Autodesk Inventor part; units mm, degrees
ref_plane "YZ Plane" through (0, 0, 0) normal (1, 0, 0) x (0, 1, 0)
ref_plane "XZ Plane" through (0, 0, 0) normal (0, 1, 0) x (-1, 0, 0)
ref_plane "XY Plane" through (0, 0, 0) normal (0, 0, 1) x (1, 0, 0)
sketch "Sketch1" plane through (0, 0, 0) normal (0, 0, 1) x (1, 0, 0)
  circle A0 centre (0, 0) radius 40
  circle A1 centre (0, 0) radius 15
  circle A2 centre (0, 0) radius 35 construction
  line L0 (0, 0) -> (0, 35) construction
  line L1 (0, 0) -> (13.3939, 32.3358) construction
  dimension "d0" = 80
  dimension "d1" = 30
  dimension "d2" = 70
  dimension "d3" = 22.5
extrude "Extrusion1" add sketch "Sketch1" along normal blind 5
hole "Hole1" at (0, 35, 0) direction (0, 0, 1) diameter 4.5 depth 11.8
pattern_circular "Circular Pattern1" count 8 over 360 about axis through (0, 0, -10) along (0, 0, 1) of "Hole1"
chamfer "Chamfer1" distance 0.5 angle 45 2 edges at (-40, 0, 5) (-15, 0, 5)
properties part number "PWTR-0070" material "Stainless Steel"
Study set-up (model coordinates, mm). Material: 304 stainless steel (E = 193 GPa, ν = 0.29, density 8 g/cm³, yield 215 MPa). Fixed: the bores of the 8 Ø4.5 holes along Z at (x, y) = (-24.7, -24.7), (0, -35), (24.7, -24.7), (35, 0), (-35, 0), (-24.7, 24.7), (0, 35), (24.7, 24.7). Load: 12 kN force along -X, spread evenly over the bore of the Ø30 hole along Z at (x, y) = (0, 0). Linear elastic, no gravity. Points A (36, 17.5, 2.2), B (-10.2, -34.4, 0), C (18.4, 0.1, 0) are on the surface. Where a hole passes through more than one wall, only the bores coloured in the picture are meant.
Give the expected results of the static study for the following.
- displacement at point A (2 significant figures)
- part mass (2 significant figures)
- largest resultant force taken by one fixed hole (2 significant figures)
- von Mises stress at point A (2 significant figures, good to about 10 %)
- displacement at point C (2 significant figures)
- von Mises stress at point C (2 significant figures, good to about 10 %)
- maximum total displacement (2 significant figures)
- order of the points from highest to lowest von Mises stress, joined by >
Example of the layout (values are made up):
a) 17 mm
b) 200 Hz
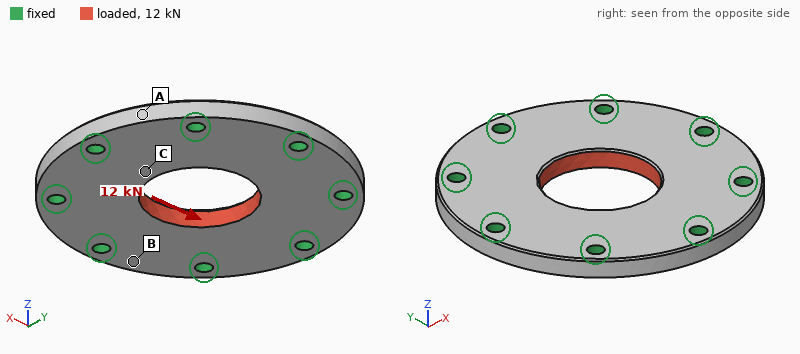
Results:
a) 1.3 µm
b) 170 g
c) 2.3 kN
d) 15 MPa
e) 2.8 µm
f) 30 MPa
g) 3.4 µm
h) C > A > B
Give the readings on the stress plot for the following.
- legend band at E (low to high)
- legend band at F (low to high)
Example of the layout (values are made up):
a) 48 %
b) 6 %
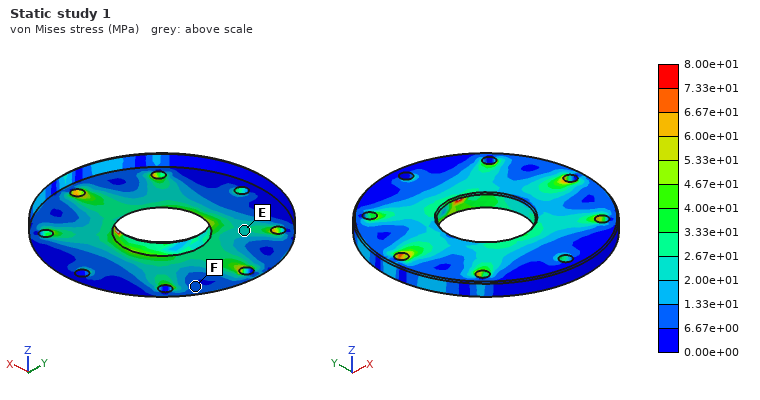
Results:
a) 2.00e+01 to 2.67e+01 MPa
b) 6.67e+00 to 1.33e+01 MPa
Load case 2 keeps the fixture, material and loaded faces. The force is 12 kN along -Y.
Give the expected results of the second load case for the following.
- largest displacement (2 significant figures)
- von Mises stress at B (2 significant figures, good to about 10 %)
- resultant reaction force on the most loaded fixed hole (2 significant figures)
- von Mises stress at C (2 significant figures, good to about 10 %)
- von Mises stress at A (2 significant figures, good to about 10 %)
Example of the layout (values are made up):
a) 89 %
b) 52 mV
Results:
a) 3.4 µm
b) 7.6 MPa
c) 2.3 kN
d) 25 MPa
e) 6.5 MPa
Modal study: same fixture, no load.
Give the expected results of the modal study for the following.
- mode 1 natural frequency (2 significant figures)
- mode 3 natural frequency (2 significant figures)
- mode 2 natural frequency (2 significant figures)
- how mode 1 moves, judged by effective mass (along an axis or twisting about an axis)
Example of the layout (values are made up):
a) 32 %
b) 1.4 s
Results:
a) 12 kHz
b) 16 kHz
c) 16 kHz
d) along Z
